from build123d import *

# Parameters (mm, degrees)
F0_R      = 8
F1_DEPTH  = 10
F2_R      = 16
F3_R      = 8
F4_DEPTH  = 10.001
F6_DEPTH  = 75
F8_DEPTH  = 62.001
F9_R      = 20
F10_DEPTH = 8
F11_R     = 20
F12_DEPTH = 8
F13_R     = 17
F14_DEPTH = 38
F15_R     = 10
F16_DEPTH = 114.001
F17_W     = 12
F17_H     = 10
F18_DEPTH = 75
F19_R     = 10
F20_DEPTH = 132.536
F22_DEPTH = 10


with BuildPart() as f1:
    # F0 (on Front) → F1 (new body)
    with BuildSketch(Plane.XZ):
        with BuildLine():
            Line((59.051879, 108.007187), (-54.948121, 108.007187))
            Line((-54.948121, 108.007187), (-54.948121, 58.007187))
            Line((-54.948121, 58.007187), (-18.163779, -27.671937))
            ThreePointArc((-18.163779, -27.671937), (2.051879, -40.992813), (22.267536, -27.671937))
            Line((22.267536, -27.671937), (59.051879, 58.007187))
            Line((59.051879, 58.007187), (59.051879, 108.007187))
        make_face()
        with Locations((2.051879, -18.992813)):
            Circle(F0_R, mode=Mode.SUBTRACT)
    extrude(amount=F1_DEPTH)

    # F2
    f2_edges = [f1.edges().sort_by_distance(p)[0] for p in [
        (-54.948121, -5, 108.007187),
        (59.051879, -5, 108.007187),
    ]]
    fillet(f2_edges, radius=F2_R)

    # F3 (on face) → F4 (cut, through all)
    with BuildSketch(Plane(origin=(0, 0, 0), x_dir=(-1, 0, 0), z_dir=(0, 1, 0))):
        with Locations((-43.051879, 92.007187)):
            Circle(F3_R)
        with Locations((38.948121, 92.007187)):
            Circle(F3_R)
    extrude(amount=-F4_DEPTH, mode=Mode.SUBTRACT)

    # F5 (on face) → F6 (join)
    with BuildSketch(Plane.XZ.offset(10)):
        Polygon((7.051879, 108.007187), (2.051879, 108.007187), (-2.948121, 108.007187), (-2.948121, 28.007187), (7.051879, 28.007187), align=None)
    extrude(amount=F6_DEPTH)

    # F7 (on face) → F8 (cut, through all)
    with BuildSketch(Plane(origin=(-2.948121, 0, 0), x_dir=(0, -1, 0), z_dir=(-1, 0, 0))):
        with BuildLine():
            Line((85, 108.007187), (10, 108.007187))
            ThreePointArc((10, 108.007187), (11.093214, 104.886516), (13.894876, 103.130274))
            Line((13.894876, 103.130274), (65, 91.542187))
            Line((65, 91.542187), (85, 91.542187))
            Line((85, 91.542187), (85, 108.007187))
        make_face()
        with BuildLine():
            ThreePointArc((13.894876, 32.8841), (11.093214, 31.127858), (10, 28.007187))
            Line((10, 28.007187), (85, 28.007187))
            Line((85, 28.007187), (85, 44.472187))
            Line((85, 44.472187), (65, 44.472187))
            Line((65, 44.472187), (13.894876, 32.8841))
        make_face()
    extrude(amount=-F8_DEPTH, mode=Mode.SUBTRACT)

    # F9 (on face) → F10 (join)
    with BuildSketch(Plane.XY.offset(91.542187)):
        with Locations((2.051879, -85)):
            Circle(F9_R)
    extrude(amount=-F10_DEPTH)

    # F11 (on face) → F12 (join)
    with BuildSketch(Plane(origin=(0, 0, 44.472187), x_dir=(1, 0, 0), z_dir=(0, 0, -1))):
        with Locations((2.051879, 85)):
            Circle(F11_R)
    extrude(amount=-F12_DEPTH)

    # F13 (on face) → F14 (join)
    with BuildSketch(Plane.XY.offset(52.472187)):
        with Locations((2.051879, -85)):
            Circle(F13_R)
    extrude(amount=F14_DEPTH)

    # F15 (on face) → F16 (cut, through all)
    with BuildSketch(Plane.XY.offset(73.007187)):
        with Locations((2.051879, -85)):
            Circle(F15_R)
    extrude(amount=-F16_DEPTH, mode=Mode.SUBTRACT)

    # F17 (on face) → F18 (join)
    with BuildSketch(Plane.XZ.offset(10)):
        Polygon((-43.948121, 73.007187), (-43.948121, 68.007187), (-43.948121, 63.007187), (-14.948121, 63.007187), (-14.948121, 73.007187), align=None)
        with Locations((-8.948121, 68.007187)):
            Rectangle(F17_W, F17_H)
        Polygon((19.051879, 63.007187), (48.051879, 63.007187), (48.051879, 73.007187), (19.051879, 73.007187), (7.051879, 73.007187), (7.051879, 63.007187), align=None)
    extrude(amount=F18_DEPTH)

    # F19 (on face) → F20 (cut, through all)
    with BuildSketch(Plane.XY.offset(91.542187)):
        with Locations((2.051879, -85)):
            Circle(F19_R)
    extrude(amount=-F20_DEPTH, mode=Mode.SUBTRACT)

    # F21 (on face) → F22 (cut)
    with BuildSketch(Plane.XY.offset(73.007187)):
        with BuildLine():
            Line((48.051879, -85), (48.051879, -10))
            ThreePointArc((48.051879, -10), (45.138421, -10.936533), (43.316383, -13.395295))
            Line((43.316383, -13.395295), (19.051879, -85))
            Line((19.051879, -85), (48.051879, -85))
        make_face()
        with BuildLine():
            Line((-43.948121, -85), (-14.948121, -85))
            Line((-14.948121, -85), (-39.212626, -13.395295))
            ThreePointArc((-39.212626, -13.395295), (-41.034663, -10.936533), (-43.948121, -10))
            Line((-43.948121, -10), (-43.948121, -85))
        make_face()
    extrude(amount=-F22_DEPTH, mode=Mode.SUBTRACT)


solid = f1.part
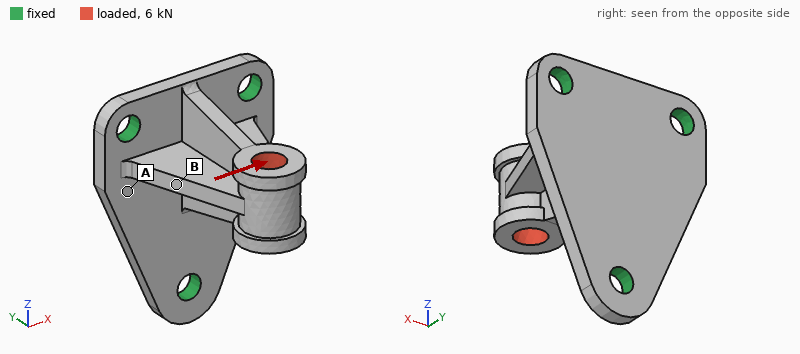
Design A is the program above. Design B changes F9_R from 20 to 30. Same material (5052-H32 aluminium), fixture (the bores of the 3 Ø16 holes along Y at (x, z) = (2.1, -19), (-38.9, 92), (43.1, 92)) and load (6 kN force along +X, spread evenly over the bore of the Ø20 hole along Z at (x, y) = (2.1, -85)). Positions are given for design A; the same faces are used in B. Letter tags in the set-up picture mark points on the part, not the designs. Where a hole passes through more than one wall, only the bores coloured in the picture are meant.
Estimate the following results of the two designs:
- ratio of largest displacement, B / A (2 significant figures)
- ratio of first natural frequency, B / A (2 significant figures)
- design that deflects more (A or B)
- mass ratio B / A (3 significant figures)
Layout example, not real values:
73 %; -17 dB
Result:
1.1; 0.90; B; 1.05
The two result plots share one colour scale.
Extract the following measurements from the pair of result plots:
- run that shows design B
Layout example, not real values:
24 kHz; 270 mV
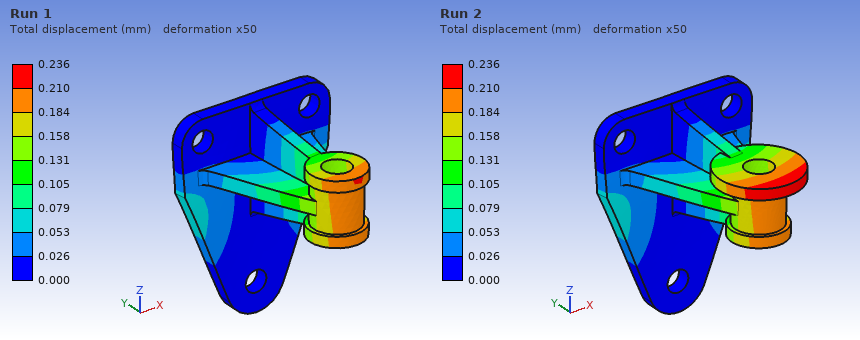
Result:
Run 2
